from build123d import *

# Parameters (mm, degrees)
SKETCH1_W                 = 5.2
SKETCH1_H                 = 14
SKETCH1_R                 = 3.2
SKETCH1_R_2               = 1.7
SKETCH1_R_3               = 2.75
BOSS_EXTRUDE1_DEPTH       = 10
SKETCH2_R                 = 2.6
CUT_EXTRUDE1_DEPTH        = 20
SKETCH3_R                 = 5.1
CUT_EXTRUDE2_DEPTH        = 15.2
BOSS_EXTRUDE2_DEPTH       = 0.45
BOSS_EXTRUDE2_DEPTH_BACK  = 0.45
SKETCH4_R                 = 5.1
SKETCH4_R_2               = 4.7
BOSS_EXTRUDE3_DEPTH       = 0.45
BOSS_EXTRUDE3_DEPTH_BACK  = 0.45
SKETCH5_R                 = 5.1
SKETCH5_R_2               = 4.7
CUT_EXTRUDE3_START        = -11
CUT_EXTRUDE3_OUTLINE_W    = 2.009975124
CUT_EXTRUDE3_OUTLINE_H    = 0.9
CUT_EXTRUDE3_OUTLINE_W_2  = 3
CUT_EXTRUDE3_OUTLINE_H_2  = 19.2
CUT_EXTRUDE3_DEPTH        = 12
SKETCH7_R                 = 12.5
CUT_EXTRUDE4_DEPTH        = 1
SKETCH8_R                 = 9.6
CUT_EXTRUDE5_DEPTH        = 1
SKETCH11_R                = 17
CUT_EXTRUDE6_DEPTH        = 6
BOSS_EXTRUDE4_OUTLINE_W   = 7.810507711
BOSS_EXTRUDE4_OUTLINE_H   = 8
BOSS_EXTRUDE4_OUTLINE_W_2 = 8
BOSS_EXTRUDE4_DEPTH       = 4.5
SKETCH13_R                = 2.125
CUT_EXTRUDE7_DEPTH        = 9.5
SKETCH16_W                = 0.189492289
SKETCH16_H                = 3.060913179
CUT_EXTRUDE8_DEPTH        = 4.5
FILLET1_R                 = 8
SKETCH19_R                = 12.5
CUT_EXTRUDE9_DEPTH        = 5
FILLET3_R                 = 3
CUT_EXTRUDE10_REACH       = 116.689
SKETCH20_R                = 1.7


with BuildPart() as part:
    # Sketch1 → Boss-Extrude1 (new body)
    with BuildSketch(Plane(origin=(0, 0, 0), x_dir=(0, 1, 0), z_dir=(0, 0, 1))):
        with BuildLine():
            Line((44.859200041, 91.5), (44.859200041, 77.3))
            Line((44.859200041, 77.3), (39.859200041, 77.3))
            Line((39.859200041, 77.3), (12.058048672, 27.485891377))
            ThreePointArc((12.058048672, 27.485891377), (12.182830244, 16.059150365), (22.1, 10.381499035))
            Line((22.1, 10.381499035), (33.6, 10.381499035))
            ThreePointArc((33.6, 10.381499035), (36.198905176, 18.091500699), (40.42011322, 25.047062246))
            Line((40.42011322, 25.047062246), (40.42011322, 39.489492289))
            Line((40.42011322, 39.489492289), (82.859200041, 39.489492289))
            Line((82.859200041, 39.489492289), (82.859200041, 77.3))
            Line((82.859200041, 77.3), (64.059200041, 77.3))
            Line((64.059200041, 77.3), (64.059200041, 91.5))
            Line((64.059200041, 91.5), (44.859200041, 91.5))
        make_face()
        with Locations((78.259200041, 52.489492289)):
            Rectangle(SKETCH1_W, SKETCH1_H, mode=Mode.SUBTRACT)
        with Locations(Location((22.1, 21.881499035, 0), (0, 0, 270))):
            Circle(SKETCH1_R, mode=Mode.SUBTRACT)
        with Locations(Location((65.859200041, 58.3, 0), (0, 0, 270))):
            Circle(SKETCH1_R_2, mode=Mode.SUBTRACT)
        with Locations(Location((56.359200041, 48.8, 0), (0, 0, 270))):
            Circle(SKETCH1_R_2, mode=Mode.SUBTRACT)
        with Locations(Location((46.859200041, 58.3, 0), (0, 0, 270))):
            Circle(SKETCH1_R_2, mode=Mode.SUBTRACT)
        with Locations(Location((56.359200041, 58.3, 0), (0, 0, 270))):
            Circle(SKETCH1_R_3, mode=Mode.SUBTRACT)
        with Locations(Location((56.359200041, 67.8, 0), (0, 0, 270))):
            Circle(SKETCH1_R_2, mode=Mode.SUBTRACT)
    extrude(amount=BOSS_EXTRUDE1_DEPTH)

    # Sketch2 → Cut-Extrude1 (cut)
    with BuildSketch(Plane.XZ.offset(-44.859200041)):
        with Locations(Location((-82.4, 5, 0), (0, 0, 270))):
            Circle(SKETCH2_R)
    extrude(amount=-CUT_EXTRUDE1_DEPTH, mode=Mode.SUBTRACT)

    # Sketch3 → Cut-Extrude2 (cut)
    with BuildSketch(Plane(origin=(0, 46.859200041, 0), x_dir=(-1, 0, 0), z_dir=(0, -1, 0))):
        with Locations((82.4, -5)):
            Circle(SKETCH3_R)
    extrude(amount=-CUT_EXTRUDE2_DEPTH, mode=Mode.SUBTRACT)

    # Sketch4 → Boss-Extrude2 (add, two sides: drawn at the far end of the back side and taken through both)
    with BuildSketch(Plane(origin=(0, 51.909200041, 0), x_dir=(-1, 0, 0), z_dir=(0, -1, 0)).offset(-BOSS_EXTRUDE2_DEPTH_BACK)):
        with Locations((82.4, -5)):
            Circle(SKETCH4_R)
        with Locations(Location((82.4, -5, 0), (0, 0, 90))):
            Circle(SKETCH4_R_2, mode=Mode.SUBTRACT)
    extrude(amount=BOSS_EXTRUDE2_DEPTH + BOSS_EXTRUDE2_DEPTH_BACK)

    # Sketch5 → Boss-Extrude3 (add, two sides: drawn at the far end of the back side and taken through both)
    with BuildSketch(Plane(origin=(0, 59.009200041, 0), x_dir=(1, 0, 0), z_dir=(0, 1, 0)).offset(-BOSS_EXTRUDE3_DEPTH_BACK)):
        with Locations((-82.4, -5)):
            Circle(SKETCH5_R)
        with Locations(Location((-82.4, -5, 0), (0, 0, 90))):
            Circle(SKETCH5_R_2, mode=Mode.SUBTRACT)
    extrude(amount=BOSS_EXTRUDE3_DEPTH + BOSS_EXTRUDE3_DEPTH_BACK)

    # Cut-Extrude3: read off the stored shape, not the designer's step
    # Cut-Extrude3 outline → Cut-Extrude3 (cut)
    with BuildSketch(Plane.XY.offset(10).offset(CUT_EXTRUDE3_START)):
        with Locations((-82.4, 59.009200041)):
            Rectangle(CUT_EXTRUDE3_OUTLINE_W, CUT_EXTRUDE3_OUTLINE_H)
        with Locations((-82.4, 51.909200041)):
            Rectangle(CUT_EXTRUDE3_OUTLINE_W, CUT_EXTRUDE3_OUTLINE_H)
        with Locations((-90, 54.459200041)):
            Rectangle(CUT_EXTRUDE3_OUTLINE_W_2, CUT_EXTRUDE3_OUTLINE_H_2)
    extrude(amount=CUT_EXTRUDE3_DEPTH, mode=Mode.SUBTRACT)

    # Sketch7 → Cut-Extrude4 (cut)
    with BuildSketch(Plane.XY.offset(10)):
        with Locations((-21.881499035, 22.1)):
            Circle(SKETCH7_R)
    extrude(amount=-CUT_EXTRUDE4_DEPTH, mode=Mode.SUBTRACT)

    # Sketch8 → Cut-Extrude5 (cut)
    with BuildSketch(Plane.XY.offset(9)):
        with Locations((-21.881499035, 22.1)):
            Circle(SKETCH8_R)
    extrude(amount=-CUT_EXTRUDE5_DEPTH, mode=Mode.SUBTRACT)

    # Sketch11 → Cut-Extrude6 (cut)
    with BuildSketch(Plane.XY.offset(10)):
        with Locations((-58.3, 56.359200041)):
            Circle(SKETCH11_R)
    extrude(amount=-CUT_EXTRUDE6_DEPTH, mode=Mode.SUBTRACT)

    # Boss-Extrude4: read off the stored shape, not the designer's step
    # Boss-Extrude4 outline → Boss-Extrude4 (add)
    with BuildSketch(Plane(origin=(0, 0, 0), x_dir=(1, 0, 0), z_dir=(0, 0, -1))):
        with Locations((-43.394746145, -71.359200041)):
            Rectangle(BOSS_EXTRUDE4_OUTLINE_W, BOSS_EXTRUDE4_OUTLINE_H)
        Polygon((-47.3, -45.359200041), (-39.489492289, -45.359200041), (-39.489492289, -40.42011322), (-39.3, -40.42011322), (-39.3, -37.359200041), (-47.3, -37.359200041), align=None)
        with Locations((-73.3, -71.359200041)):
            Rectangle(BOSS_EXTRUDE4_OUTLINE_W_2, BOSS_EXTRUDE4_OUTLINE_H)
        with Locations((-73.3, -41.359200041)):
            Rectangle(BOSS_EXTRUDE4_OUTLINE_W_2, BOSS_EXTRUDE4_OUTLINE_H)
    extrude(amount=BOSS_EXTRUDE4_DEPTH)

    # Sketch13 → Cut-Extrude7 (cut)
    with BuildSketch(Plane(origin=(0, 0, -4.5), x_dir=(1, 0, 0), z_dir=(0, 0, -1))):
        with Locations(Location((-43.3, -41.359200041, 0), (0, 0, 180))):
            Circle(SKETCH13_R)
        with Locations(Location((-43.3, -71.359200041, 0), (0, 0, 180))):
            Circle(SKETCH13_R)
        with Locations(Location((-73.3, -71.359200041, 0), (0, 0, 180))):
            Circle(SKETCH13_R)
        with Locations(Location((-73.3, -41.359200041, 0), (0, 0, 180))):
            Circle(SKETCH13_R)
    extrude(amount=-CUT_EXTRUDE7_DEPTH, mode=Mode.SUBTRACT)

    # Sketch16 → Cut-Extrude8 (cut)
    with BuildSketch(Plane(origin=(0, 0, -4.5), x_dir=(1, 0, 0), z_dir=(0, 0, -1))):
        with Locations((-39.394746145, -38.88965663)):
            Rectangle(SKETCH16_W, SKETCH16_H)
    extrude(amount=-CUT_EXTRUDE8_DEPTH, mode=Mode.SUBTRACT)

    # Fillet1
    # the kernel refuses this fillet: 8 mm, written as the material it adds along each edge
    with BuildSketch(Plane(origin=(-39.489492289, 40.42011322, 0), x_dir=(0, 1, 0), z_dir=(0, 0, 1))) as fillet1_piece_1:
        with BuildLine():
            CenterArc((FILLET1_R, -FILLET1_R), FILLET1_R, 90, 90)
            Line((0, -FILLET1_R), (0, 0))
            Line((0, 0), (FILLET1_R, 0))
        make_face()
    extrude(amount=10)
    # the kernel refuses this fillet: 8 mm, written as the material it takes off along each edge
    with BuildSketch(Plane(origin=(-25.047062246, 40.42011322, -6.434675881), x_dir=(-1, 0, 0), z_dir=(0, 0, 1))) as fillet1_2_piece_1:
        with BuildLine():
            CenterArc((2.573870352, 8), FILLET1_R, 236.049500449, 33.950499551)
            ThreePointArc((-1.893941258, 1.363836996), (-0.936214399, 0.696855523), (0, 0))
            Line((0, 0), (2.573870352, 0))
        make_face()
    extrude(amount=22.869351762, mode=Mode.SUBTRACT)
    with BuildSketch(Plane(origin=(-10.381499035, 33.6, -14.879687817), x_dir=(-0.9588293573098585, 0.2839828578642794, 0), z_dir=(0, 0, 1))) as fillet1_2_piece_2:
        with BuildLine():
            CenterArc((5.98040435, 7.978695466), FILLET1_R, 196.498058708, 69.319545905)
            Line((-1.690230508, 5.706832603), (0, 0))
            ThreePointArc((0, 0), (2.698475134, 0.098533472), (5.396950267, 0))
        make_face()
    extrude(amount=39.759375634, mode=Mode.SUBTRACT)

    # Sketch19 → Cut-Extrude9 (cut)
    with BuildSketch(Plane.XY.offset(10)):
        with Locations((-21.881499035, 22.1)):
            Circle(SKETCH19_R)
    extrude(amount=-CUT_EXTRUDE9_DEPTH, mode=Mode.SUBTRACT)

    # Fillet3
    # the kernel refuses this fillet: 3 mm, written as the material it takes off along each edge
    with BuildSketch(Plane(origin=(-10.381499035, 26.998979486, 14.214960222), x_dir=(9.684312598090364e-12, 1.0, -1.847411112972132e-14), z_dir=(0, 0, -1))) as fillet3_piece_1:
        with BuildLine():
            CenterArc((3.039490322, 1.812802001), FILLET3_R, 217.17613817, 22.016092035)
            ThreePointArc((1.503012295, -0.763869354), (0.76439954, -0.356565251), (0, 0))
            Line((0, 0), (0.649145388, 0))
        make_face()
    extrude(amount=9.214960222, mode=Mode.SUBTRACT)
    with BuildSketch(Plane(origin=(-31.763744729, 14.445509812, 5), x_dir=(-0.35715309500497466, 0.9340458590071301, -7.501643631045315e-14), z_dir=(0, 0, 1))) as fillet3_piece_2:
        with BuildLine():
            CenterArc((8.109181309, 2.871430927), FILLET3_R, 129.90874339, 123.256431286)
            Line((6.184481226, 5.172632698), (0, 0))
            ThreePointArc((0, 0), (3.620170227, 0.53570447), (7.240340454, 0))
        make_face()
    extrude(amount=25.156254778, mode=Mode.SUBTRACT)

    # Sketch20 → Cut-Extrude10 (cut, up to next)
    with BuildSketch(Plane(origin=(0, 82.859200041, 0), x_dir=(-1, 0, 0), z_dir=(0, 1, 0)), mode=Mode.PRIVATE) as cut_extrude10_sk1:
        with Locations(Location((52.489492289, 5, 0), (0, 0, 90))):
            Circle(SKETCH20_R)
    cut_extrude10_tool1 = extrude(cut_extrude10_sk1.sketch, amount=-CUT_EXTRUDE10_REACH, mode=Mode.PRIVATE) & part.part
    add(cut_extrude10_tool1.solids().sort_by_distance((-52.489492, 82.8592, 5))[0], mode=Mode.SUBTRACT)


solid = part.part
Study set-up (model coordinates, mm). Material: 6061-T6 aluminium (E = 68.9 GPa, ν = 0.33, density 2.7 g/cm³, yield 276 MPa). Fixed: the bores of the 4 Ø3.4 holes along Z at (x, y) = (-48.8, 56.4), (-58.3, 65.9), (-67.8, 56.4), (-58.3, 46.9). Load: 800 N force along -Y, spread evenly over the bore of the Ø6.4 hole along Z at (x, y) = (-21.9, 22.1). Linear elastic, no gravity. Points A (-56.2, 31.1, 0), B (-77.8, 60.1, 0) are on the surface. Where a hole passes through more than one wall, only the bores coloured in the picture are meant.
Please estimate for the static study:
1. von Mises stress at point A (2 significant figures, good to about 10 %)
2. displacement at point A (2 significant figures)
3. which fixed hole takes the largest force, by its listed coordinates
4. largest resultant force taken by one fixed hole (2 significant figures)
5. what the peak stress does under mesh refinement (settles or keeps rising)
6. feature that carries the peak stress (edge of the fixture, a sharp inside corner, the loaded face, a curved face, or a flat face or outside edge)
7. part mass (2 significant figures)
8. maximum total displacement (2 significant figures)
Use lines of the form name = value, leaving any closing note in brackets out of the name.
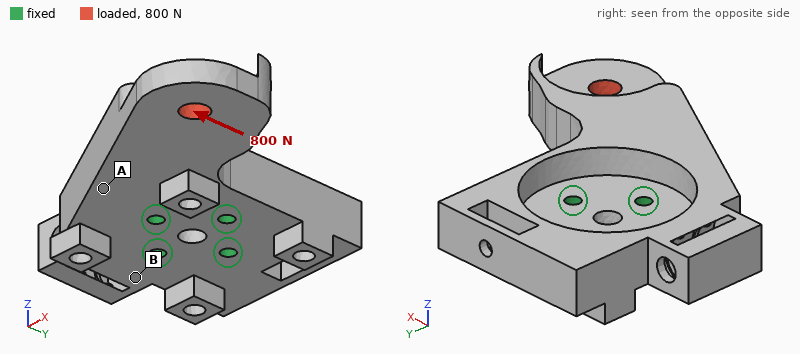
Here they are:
von Mises stress at point A = 19 MPa
displacement at point A = 9.6 µm
which fixed hole takes the largest force, by its listed coordinates = (-48.8, 56.4)
largest resultant force taken by one fixed hole = 1.3 kN
what the peak stress does under mesh refinement = keeps rising
feature that carries the peak stress = edge of the fixture
part mass = 54 g
maximum total displacement = 60 µm
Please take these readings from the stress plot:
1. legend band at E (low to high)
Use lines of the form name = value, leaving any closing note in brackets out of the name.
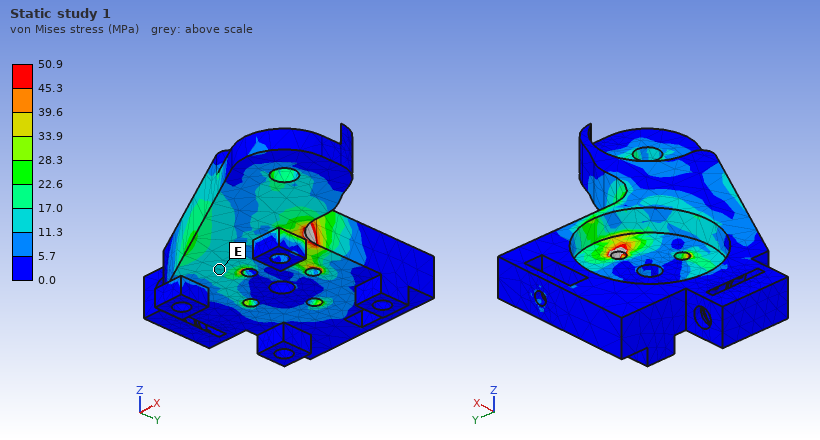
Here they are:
legend band at E = 11.3 to 17.0 MPa
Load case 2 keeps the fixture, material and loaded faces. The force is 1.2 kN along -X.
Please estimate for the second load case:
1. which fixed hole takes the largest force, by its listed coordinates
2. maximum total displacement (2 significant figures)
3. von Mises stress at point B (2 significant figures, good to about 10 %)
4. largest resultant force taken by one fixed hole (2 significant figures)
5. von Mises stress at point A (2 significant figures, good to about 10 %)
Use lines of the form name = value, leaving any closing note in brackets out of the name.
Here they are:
which fixed hole takes the largest force, by its listed coordinates = (-58.3, 46.9)
maximum total displacement = 69 µm
von Mises stress at point B = 7.0 MPa
largest resultant force taken by one fixed hole = 1.5 kN
von Mises stress at point A = 28 MPa
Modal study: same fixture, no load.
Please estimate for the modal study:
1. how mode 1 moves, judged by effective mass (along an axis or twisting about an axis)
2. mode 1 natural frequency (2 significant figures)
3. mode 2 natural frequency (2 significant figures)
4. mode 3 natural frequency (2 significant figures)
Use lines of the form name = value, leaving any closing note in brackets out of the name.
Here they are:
how mode 1 moves, judged by effective mass = along Z
mode 1 natural frequency = 2100 Hz
mode 2 natural frequency = 6200 Hz
mode 3 natural frequency = 6700 Hz
